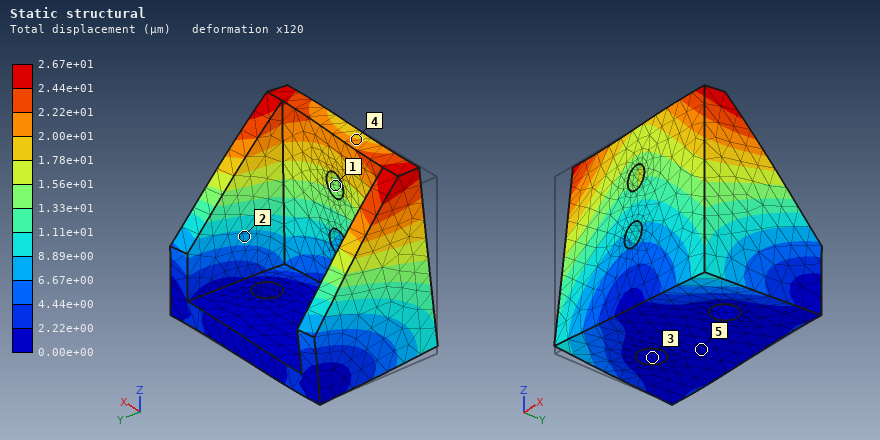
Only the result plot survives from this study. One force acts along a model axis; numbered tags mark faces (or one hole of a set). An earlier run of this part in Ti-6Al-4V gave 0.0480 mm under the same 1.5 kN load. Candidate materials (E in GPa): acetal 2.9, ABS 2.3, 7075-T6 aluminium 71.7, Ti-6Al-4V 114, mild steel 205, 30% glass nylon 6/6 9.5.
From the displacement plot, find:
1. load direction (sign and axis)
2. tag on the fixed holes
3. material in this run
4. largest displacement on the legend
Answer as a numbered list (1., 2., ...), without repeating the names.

1. +X
2. 3
3. mild steel
4. 2.67e+01 µm
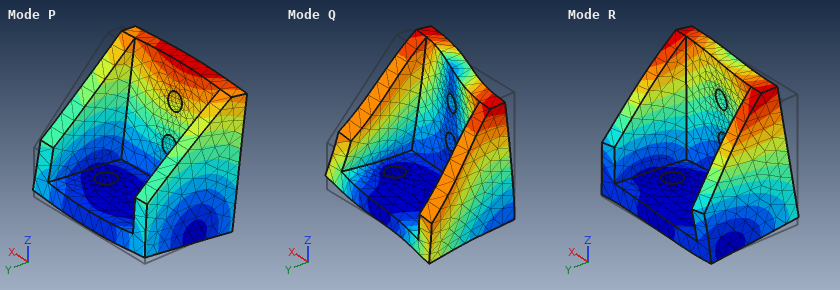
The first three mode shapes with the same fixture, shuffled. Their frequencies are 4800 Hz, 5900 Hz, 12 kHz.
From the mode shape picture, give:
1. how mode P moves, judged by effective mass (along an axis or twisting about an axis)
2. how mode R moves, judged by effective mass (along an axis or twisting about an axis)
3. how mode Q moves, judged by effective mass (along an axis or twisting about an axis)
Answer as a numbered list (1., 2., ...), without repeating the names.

1. along Y
2. along X
3. along X
